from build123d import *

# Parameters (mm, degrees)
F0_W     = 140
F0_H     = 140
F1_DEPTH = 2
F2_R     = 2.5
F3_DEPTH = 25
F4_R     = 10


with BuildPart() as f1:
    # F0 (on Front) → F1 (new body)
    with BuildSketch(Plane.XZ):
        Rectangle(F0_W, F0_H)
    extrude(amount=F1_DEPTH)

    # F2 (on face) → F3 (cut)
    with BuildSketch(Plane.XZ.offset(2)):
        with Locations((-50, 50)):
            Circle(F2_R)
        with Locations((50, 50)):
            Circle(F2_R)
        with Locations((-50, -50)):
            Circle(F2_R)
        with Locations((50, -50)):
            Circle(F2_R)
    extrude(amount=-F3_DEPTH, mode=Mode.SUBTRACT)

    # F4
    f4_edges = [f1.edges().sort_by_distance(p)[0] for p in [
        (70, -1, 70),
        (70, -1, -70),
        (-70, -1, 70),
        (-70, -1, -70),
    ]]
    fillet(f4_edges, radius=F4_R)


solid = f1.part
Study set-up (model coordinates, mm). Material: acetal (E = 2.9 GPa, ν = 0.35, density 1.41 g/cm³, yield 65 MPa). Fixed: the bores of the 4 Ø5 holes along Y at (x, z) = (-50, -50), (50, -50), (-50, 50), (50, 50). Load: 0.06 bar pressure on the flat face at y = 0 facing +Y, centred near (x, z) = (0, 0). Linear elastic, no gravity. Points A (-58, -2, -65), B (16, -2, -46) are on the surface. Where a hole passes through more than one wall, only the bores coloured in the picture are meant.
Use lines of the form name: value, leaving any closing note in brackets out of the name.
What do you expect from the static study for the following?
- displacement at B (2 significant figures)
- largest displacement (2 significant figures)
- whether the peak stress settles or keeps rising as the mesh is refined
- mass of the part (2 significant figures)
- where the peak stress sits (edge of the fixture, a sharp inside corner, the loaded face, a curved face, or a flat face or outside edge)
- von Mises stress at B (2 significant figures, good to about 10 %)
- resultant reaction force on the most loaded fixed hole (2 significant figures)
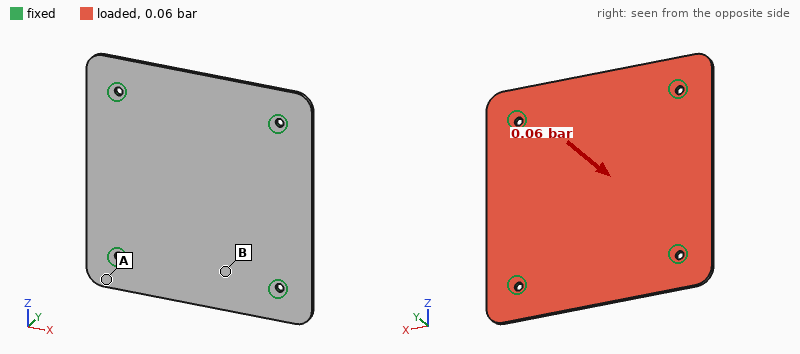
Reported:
displacement at B: 0.93 mm
largest displacement: 1.8 mm
whether the peak stress settles or keeps rising as the mesh is refined: keeps rising
mass of the part: 55 g
where the peak stress sits: edge of the fixture
von Mises stress at B: 3.5 MPa
resultant reaction force on the most loaded fixed hole: 29 N
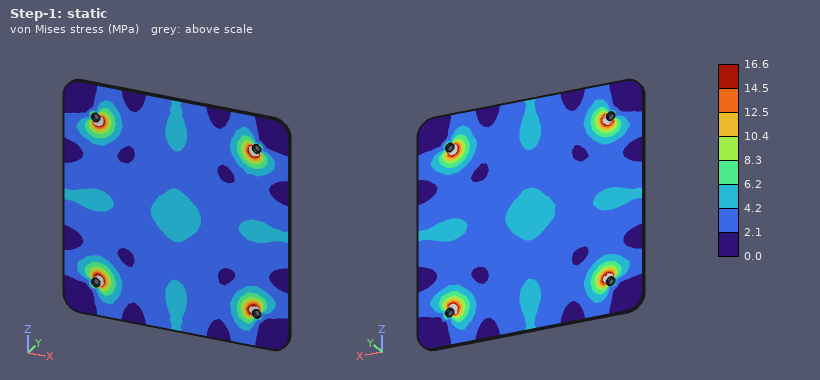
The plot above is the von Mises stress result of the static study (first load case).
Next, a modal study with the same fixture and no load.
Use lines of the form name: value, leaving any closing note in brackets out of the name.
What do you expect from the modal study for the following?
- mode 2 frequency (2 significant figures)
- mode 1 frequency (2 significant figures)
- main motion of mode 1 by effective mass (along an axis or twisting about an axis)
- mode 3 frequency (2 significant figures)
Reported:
mode 2 frequency: 310 Hz
mode 1 frequency: 210 Hz
main motion of mode 1 by effective mass: along Y
mode 3 frequency: 310 Hz
